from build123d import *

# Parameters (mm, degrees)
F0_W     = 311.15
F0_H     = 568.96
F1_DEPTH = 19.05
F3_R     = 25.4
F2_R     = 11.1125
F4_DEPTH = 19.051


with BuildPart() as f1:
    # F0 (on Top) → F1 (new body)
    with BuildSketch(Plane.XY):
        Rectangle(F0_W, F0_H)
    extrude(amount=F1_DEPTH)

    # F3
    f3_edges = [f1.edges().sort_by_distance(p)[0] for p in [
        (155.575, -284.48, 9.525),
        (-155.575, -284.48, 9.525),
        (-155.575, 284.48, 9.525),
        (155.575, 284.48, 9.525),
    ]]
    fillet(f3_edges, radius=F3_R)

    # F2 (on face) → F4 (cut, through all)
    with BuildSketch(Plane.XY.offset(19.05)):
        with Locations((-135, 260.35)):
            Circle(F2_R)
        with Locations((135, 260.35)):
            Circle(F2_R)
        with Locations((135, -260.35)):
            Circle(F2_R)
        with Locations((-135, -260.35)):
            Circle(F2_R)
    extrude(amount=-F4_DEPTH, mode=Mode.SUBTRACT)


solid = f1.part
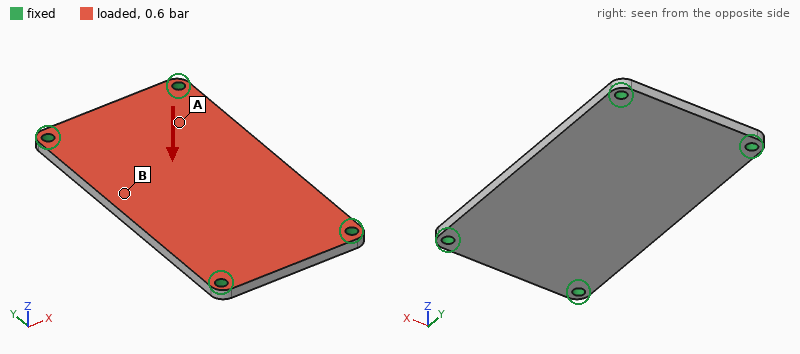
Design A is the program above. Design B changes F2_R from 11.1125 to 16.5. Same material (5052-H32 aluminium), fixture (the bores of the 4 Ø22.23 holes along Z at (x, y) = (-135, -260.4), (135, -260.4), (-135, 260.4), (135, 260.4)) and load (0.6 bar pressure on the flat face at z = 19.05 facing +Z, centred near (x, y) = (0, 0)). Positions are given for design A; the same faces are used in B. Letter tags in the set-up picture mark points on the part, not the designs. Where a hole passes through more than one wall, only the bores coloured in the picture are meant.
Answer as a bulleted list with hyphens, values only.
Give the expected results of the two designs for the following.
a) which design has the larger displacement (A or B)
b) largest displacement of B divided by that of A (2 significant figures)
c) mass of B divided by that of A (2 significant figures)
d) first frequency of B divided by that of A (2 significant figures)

- A
- 0.87
- 0.99
- 1.1
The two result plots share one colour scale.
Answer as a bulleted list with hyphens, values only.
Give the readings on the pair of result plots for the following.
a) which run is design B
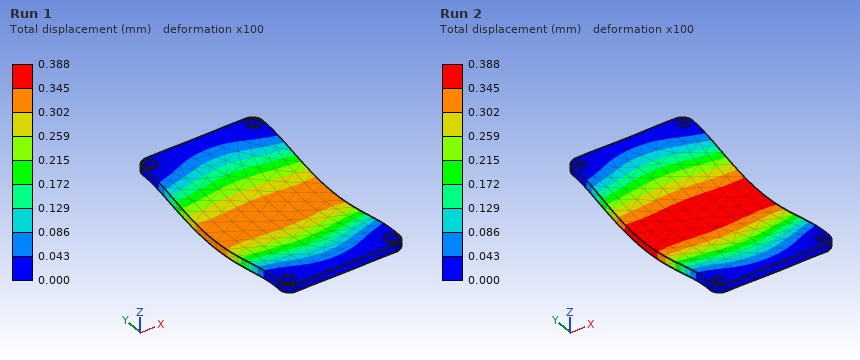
- Run 1
